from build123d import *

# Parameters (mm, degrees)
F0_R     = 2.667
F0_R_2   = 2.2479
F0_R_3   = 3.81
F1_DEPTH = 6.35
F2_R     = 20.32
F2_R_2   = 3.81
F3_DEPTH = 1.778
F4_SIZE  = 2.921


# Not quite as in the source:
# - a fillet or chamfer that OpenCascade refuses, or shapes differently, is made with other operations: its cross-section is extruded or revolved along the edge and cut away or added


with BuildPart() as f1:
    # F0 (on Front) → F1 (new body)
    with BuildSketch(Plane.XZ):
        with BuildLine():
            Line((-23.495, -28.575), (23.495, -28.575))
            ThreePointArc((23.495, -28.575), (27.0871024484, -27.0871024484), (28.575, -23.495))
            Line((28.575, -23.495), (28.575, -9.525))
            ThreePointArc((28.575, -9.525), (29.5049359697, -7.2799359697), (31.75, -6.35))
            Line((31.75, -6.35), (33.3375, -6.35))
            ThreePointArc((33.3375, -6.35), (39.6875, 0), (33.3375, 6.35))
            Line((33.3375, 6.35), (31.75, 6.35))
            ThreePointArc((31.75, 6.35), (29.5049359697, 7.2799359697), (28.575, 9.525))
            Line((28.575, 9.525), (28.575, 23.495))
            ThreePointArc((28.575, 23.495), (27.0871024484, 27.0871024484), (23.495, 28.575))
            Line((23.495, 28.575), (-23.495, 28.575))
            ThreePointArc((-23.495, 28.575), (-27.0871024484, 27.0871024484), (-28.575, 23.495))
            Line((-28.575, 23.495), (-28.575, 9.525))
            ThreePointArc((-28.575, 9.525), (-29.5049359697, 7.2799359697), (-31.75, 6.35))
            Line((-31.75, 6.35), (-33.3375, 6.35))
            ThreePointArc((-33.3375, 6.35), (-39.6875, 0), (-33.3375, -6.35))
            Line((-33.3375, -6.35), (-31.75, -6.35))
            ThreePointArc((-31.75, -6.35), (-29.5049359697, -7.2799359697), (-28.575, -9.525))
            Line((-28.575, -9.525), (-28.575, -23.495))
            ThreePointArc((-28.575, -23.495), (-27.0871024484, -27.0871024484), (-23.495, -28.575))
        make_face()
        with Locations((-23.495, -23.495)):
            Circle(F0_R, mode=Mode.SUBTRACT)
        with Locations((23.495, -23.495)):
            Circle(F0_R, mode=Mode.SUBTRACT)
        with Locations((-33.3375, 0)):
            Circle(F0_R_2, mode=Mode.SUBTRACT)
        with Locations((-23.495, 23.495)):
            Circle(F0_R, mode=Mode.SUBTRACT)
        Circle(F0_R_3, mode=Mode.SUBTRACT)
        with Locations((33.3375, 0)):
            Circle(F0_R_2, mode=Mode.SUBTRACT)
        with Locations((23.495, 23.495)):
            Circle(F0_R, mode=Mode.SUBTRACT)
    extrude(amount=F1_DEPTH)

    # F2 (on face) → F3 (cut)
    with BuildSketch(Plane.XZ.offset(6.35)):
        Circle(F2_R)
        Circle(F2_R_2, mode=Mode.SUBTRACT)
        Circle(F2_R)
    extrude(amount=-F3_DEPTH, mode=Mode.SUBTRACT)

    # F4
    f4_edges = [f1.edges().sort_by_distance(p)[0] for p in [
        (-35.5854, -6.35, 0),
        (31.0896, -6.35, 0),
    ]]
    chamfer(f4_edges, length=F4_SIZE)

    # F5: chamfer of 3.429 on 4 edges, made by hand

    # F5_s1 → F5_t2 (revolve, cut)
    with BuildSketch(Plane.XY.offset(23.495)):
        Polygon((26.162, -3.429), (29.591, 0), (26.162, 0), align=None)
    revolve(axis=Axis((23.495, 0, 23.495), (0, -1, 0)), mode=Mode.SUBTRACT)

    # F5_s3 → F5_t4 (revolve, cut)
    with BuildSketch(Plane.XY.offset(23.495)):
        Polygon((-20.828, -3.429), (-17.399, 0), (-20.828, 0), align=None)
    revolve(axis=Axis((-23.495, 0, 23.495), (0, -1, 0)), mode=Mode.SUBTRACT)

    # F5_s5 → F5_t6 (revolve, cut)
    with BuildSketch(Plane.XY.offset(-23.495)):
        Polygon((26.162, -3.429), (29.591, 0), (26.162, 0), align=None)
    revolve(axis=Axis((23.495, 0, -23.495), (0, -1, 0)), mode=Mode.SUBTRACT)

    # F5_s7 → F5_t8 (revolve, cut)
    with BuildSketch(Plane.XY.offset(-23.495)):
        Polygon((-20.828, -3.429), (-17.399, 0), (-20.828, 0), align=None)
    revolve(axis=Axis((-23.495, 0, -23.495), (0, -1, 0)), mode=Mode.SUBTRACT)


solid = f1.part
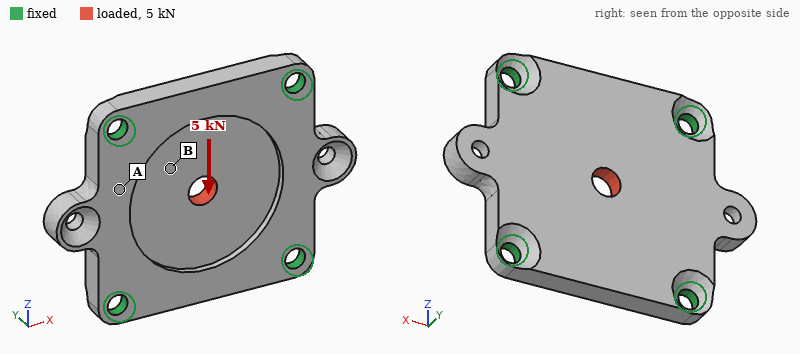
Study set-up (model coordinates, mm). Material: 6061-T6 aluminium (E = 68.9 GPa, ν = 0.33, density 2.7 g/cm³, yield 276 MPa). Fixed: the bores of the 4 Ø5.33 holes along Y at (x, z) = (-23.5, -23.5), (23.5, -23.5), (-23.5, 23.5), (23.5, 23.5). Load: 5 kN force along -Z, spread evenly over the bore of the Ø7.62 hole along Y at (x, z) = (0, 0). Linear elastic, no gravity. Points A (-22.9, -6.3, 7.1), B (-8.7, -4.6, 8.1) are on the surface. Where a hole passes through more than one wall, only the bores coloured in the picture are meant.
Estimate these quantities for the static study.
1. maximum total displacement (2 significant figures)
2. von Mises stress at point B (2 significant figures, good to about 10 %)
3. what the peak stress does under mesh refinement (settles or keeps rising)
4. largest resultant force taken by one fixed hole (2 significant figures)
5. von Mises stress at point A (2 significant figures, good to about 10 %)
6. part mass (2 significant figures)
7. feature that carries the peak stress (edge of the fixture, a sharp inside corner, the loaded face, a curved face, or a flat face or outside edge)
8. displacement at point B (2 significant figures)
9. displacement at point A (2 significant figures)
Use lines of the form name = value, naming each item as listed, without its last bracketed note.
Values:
maximum total displacement = 14 µm
von Mises stress at point B = 26 MPa
what the peak stress does under mesh refinement = keeps rising
largest resultant force taken by one fixed hole = 1.4 kN
von Mises stress at point A = 11 MPa
part mass = 49 g
feature that carries the peak stress = edge of the fixture
displacement at point B = 8.9 µm
displacement at point A = 3.5 µm
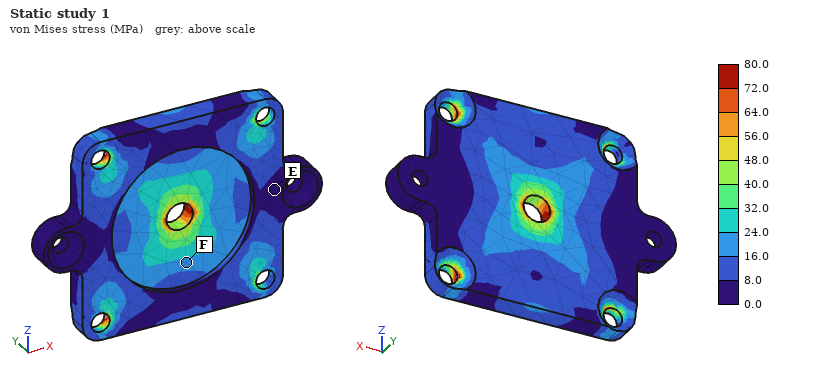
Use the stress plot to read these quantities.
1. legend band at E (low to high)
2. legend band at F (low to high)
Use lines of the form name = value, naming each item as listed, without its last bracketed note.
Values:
legend band at E = 0.0 to 8.0 MPa
legend band at F = 16.0 to 24.0 MPa
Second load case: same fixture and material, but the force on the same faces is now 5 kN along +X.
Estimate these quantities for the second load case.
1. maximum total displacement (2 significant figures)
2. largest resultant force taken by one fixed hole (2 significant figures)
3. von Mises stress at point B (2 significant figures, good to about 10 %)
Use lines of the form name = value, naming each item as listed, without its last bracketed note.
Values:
maximum total displacement = 14 µm
largest resultant force taken by one fixed hole = 1.4 kN
von Mises stress at point B = 26 MPa
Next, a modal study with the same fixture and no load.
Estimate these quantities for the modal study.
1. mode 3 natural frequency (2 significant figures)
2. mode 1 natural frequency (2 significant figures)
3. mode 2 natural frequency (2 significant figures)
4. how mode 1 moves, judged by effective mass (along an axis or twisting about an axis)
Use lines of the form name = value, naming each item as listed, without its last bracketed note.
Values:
mode 3 natural frequency = 9600 Hz
mode 1 natural frequency = 8300 Hz
mode 2 natural frequency = 9600 Hz
how mode 1 moves, judged by effective mass = along Y
